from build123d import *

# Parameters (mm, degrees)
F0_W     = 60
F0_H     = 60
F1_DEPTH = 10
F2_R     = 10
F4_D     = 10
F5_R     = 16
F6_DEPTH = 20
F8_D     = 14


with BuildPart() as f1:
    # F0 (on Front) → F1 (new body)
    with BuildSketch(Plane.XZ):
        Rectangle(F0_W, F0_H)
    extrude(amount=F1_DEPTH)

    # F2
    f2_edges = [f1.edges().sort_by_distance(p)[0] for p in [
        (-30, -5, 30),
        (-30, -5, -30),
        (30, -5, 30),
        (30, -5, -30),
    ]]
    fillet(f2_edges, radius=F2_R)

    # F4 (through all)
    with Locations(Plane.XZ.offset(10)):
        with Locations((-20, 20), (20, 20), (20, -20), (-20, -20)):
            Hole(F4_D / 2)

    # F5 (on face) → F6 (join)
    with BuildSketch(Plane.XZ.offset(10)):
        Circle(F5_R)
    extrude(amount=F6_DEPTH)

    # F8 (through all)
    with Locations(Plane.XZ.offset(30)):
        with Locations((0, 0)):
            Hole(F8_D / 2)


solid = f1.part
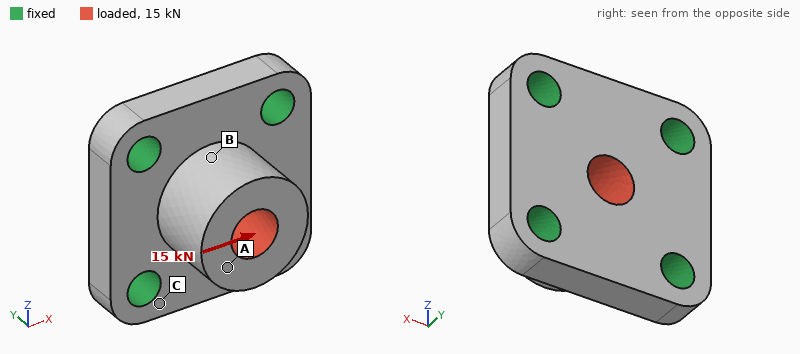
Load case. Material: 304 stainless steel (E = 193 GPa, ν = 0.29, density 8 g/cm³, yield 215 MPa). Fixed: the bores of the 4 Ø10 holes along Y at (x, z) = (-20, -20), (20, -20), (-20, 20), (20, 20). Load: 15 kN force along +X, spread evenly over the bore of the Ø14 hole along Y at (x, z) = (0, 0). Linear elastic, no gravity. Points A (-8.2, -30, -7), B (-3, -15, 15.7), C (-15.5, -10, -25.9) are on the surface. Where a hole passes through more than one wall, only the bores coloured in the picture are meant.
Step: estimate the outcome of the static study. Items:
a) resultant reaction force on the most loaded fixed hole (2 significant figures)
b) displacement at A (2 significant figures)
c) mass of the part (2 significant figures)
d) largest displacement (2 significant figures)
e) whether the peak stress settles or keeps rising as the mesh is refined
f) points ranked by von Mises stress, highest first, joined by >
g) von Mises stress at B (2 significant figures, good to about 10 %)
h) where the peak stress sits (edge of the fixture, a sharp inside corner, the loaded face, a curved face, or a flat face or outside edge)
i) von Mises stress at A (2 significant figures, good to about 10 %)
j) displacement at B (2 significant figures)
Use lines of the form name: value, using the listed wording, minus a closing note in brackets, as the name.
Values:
resultant reaction force on the most loaded fixed hole: 4.6 kN
displacement at A: 11 µm
mass of the part: 350 g
largest displacement: 12 µm
whether the peak stress settles or keeps rising as the mesh is refined: keeps rising
points ranked by von Mises stress, highest first, joined by >: B > A > C
von Mises stress at B: 24 MPa
where the peak stress sits: edge of the fixture
von Mises stress at A: 14 MPa
displacement at B: 4.6 µm
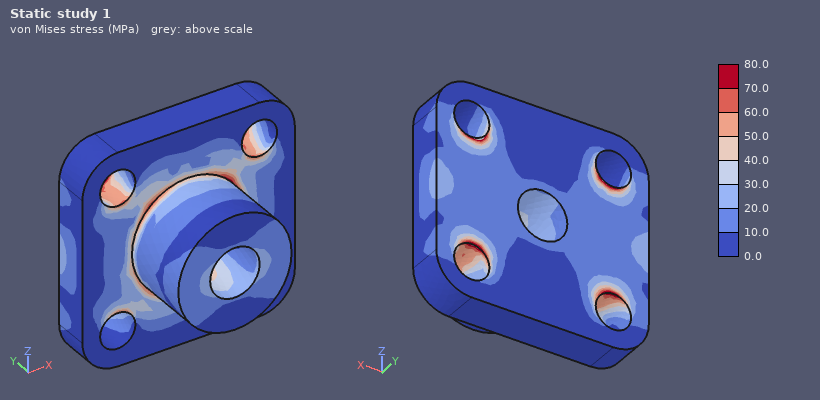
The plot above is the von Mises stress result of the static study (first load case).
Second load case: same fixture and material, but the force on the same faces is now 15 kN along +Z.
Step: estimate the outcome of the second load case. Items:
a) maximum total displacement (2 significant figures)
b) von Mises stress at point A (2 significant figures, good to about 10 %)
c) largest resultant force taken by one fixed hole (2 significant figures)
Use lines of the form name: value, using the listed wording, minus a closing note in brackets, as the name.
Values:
maximum total displacement: 12 µm
von Mises stress at point A: 12 MPa
largest resultant force taken by one fixed hole: 4.6 kN
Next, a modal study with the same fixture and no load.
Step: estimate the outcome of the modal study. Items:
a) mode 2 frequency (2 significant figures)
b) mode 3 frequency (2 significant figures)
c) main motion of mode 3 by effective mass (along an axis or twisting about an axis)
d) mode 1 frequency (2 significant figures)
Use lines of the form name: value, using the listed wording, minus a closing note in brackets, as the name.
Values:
mode 2 frequency: 16 kHz
mode 3 frequency: 19 kHz
main motion of mode 3 by effective mass: along Y
mode 1 frequency: 16 kHz
